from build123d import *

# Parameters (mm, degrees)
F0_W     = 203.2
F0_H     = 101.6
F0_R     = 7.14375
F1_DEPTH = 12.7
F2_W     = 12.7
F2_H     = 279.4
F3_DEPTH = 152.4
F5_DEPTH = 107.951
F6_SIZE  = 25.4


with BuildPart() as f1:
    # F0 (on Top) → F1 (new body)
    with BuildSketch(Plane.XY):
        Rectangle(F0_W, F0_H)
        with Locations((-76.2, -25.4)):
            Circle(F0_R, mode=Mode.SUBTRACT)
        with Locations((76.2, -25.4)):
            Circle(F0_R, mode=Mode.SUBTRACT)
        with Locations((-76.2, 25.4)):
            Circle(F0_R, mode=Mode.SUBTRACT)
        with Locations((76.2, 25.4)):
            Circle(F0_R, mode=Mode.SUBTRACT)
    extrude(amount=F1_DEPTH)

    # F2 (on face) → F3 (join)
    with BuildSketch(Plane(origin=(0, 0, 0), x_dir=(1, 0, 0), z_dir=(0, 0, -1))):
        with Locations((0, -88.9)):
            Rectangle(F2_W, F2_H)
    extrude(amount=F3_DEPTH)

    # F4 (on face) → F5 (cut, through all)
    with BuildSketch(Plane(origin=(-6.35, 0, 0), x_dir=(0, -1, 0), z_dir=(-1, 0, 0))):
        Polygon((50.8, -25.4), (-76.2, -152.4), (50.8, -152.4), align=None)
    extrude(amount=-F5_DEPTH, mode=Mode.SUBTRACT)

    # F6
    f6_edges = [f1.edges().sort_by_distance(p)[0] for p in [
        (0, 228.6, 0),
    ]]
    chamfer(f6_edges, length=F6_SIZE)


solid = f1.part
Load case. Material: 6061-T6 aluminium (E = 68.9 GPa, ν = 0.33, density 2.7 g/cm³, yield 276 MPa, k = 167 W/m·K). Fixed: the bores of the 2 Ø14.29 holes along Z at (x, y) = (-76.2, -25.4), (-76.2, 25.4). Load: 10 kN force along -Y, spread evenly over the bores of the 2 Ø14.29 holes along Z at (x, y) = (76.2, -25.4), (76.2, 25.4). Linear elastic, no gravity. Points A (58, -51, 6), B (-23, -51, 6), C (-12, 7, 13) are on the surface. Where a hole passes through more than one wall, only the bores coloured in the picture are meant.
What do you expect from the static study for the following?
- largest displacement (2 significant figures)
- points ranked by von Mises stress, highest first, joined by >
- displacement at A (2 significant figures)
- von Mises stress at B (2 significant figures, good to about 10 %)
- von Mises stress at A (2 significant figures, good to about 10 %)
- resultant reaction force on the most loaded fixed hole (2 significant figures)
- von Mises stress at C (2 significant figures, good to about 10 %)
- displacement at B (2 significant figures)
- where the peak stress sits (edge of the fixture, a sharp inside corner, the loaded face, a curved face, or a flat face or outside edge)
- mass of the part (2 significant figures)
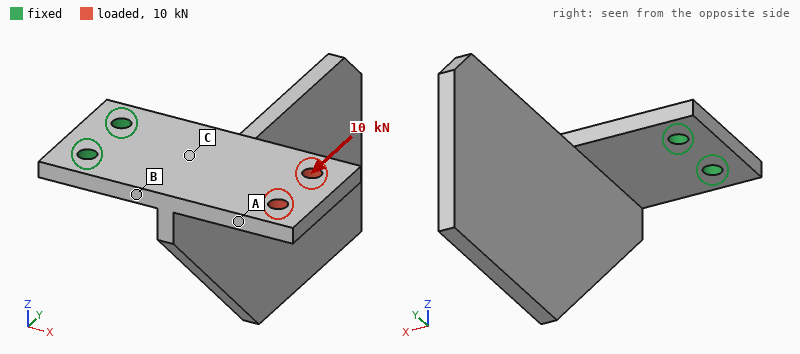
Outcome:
0.36 mm
B > C > A
0.22 mm
44 MPa
9.1 MPa
26 kN
23 MPa
0.084 mm
edge of the fixture
1.9 kg
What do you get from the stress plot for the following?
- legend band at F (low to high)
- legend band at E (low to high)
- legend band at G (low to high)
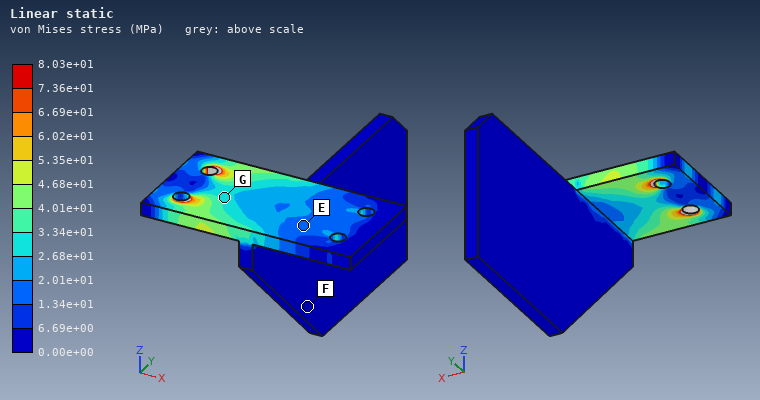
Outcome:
0.00e+00 to 6.69e+00 MPa
1.34e+01 to 2.01e+01 MPa
2.68e+01 to 3.34e+01 MPa
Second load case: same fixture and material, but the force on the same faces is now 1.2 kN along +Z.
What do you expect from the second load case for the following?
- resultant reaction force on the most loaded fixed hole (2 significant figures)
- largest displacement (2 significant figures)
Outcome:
600 N
1.3 mm
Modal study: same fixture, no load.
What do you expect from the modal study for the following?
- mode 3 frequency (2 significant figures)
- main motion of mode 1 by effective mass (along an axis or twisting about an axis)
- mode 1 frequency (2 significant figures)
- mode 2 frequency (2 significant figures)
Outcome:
300 Hz
along X
130 Hz
200 Hz
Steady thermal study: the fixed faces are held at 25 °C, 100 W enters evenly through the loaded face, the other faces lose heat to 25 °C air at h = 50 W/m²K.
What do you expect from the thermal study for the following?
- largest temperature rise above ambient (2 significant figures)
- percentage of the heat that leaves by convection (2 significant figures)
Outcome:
43 K
63 %
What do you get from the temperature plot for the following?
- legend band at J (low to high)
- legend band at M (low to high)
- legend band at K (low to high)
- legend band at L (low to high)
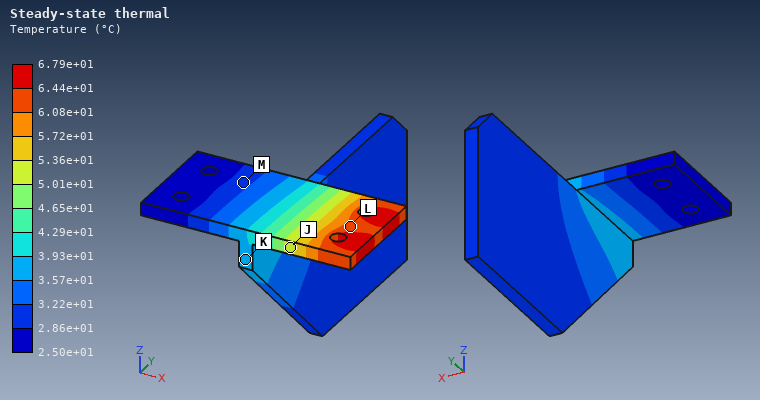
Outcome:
5.01e+01 to 5.36e+01 °C
2.86e+01 to 3.22e+01 °C
3.57e+01 to 3.93e+01 °C
6.08e+01 to 6.44e+01 °C
